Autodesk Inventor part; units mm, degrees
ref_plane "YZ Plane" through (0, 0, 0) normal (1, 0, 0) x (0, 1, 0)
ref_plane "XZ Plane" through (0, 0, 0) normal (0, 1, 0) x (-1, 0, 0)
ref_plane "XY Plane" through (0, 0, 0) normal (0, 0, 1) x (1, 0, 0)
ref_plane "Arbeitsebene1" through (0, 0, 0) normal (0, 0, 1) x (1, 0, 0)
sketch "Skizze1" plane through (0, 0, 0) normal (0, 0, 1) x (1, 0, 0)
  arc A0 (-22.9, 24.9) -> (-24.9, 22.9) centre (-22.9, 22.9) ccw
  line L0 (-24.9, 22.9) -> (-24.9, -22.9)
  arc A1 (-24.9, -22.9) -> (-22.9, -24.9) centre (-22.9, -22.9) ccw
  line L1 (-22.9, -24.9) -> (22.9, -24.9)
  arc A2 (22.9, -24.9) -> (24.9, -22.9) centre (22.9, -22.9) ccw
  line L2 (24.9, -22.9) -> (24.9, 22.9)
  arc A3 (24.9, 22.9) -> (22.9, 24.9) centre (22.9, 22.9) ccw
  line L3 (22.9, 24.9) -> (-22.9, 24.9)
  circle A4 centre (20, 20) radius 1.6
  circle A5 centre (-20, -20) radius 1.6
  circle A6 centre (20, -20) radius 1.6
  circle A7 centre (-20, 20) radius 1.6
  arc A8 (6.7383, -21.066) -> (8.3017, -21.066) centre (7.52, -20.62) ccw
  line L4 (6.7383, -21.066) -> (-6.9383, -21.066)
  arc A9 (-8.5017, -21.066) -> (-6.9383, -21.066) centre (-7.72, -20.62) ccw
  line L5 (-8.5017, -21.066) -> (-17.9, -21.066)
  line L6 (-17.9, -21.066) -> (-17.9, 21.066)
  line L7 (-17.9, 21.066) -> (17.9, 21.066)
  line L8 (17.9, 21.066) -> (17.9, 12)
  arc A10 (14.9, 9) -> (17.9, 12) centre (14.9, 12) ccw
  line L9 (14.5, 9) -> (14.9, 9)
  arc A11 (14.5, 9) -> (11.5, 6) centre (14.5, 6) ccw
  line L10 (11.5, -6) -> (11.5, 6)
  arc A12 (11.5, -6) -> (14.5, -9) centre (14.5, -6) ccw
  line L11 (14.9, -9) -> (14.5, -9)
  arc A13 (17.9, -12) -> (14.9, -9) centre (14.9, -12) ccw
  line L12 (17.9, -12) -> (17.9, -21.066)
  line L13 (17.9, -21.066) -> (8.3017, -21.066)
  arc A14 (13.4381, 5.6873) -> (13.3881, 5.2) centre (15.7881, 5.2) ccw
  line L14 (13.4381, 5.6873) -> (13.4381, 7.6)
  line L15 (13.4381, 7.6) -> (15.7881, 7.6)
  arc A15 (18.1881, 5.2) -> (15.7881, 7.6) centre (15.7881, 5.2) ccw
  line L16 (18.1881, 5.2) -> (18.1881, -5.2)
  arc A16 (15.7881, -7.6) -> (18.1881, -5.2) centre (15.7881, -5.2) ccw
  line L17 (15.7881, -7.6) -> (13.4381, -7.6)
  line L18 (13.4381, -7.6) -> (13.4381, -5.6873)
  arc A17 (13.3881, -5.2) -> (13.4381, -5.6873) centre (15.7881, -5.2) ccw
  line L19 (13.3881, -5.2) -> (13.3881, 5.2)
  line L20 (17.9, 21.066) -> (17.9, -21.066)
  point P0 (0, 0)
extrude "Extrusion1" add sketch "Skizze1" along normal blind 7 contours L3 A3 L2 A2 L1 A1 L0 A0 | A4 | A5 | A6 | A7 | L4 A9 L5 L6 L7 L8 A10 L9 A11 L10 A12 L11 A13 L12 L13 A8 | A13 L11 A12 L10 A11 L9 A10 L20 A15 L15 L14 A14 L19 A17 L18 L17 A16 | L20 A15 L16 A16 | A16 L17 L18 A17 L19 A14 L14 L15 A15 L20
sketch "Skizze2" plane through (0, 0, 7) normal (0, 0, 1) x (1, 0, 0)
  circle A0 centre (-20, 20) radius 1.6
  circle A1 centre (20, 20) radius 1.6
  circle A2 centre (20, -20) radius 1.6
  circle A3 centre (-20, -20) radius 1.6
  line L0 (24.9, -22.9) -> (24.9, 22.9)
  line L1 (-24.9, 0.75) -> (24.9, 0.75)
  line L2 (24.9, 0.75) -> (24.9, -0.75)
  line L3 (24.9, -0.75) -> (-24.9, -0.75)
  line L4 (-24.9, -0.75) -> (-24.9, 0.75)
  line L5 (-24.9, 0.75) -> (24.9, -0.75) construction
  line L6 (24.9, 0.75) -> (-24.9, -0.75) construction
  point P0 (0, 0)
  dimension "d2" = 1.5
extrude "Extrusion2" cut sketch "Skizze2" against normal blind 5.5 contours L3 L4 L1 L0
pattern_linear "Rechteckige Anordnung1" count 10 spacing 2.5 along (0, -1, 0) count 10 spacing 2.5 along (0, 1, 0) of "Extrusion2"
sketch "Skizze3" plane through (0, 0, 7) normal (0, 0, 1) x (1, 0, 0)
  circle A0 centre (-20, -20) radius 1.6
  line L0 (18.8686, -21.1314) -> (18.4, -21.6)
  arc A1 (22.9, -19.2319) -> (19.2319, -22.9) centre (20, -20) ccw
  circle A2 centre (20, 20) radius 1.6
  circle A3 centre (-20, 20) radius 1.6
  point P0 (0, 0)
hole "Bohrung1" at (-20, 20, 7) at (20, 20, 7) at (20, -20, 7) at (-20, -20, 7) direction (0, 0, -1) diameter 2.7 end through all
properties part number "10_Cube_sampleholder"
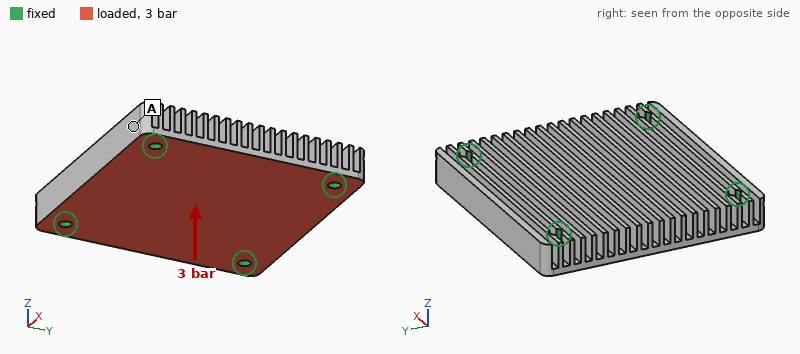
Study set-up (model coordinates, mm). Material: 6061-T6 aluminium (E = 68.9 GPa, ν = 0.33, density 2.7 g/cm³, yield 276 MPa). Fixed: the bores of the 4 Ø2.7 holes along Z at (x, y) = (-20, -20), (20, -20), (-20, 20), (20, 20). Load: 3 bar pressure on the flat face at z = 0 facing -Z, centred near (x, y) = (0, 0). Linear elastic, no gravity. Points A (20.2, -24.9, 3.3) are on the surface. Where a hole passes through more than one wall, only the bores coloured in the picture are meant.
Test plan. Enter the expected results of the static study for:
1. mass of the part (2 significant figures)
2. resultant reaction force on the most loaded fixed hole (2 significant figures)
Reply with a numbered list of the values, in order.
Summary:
1. 26 g
2. 180 N
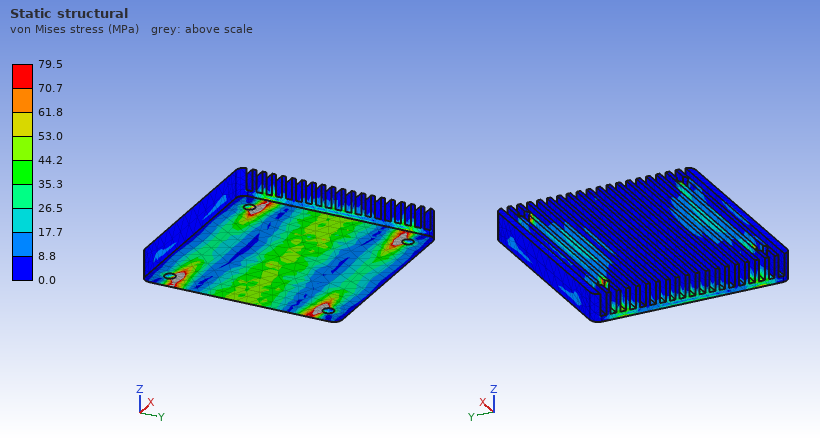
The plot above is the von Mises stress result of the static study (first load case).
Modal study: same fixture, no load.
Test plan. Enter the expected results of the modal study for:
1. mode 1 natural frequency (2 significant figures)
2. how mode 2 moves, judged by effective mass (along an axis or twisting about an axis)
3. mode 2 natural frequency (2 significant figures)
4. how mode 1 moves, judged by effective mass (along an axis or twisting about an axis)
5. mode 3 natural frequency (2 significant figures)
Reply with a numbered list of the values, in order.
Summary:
1. 3100 Hz
2. twisting about Y
3. 4100 Hz
4. along Z
5. 7800 Hz
